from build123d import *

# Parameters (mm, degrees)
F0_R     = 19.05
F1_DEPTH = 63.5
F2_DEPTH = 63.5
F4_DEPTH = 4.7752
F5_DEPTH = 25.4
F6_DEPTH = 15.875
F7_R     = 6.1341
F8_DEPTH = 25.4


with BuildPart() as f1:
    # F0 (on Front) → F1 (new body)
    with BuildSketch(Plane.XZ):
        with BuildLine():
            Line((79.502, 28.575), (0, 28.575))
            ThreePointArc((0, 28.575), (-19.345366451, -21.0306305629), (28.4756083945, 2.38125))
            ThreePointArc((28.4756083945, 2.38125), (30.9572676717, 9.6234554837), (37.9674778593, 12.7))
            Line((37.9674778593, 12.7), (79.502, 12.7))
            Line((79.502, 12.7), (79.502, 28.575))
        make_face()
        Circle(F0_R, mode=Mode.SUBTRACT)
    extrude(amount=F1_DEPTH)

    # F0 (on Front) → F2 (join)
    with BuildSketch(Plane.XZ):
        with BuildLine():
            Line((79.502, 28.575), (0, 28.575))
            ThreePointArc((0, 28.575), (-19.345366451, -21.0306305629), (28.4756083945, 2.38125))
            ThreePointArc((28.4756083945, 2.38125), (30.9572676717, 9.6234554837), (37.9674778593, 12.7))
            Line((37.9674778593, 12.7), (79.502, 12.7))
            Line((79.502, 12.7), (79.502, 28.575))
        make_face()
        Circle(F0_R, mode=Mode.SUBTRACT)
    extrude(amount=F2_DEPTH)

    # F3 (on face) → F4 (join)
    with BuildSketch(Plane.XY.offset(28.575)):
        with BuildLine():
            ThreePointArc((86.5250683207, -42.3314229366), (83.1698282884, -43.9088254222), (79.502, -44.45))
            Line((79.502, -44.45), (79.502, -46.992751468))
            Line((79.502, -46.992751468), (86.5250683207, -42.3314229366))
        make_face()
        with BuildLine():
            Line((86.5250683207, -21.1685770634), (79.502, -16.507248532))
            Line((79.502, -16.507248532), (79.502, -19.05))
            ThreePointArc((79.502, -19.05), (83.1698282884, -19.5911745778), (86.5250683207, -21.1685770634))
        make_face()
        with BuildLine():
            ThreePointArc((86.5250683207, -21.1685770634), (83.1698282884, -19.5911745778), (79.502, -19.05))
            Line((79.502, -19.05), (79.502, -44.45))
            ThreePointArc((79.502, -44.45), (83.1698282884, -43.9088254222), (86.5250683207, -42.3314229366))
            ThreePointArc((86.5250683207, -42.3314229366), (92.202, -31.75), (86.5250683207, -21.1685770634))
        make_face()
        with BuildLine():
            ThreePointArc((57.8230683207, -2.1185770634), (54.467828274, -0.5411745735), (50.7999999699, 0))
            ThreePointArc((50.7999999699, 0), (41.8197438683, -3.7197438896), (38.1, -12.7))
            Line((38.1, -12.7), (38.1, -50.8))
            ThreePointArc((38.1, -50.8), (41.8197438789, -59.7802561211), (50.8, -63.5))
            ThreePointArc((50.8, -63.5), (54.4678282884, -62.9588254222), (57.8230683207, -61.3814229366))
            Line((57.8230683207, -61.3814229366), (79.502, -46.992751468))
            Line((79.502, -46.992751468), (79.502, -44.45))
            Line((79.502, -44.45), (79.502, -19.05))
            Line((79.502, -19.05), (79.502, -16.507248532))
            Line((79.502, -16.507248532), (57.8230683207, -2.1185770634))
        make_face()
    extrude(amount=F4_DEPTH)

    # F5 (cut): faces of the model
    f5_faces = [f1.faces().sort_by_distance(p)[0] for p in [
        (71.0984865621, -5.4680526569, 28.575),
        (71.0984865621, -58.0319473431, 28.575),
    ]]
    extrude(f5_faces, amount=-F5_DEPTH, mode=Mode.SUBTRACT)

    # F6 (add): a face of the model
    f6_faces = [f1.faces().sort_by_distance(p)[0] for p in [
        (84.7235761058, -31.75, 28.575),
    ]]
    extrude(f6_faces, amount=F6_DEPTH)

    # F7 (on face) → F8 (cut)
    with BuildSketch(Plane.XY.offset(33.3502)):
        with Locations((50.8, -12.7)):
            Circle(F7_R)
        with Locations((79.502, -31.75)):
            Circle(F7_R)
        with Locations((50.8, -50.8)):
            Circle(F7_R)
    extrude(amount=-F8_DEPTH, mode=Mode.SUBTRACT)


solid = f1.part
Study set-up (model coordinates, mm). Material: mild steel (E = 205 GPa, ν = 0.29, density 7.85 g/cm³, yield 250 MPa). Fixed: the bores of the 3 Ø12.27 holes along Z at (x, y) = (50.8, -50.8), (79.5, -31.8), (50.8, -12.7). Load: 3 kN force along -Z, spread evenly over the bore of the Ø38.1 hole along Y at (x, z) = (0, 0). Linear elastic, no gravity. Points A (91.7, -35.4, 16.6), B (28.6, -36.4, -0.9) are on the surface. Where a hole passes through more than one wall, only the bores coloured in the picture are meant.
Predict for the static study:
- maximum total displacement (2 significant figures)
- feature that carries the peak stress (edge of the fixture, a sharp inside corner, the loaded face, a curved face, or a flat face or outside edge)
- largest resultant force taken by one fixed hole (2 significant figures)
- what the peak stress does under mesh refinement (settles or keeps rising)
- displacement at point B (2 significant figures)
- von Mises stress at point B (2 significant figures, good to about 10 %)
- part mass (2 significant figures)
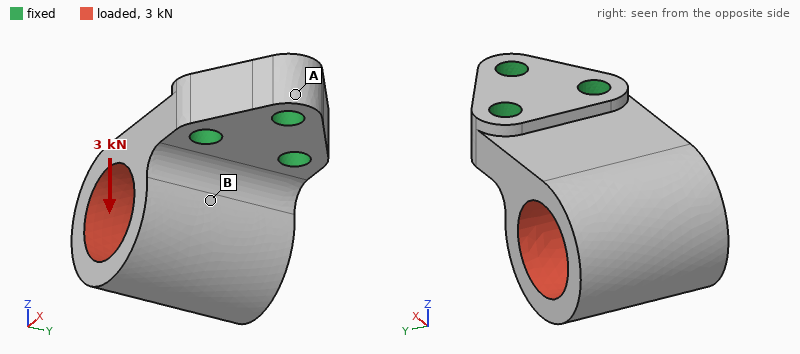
44 µm
edge of the fixture
1.7 kN
keeps rising
12 µm
9.7 MPa
1.2 kg
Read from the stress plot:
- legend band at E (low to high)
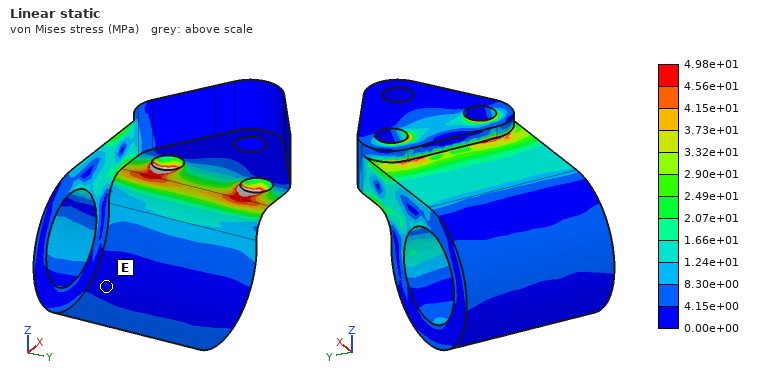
0.00e+00 to 4.15e+00 MPa
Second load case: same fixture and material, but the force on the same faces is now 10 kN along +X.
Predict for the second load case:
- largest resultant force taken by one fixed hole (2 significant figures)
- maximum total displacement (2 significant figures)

4.8 kN
89 µm
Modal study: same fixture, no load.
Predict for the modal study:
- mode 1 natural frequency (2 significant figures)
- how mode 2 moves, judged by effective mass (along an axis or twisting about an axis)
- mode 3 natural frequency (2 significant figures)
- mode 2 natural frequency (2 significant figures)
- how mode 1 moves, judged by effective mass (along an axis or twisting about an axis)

1600 Hz
along Y
6100 Hz
3800 Hz
along Z
